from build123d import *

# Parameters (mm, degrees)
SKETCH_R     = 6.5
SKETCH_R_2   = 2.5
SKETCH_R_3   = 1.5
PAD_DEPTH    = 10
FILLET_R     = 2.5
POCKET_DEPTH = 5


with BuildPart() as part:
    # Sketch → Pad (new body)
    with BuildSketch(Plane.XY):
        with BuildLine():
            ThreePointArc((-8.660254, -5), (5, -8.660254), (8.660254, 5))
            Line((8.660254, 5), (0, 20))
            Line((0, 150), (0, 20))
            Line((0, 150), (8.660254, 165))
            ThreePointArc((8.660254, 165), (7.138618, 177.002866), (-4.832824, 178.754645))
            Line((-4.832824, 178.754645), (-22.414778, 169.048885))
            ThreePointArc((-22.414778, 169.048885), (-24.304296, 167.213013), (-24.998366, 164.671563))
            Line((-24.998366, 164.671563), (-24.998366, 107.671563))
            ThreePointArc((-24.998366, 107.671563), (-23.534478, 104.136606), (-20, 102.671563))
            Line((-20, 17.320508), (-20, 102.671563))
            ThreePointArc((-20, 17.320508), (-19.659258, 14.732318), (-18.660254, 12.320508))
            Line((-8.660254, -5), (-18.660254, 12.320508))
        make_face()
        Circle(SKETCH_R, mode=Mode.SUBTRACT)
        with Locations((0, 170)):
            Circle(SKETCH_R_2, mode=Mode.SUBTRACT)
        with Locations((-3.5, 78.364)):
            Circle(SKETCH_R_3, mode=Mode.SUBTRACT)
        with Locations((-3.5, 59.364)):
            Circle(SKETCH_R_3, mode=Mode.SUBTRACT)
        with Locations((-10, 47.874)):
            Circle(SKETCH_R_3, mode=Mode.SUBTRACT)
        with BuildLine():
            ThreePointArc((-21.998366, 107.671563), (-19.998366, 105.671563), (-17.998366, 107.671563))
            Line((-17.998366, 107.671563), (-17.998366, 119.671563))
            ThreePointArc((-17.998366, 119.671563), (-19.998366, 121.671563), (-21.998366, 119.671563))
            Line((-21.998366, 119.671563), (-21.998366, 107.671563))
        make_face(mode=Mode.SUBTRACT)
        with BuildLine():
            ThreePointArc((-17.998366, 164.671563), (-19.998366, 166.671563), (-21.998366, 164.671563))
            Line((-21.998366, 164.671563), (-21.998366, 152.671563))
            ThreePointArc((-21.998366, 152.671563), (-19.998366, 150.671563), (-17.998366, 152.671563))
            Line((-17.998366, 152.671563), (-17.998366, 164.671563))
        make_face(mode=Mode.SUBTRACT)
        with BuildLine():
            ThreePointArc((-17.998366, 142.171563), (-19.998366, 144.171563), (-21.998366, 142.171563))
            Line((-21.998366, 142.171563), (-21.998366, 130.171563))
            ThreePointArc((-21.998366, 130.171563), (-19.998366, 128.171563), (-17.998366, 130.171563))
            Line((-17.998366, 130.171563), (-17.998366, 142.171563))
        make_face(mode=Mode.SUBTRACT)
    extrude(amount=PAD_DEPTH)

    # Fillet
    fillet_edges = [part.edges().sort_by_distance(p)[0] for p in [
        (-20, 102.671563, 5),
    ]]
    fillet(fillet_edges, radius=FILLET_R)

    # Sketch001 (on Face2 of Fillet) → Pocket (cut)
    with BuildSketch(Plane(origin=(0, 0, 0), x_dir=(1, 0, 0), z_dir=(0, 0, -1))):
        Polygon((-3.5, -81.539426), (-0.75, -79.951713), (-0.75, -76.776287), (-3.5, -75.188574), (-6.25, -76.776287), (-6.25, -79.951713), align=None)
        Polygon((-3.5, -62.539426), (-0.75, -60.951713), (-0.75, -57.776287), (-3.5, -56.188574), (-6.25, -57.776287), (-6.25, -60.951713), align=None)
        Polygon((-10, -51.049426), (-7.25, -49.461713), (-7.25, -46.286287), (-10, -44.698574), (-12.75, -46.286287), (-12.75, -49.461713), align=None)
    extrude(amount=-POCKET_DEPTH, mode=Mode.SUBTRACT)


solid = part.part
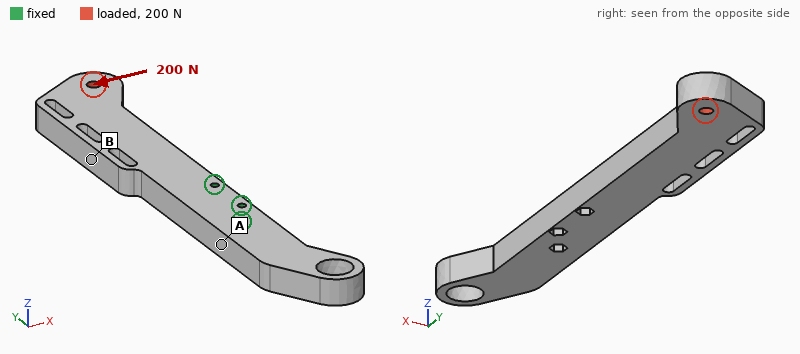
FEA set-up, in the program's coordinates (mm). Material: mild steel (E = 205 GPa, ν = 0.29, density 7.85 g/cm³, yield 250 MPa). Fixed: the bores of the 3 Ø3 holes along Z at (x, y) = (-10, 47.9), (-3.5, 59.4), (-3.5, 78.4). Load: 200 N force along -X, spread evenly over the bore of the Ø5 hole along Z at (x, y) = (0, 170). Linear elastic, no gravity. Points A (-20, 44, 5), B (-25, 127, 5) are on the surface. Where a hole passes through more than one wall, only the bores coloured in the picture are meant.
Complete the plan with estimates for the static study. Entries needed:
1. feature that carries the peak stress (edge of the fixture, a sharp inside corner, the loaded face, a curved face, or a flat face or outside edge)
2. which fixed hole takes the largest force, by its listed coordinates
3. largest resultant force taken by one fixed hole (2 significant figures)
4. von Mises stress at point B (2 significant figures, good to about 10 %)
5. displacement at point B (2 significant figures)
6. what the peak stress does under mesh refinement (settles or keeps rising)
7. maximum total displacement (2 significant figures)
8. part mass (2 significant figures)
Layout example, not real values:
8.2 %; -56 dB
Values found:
edge of the fixture; (-3.5, 78.4); 1.1 kN; 12 MPa; 24 µm; keeps rising; 59 µm; 300 g
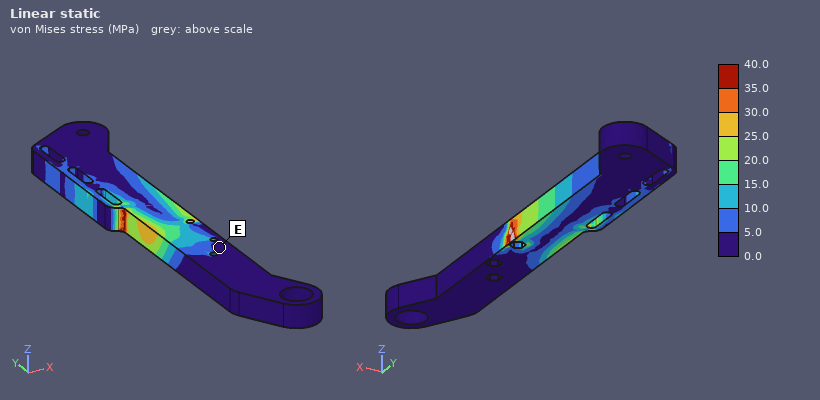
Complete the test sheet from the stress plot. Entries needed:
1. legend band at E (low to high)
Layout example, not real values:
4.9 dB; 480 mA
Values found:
0.0 to 5.0 MPa
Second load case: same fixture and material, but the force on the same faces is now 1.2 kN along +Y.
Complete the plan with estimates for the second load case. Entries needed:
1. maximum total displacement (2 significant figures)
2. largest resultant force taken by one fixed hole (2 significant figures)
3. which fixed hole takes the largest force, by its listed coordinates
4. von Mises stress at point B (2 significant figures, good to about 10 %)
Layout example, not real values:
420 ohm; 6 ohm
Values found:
48 µm; 1.2 kN; (-3.5, 78.4); 12 MPa
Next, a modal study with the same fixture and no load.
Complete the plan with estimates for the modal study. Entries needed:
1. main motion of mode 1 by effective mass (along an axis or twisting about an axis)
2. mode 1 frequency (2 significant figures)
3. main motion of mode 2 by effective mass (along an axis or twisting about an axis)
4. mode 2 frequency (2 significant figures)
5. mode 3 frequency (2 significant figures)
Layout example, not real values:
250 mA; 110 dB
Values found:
along Z; 640 Hz; along X; 1200 Hz; 2300 Hz
